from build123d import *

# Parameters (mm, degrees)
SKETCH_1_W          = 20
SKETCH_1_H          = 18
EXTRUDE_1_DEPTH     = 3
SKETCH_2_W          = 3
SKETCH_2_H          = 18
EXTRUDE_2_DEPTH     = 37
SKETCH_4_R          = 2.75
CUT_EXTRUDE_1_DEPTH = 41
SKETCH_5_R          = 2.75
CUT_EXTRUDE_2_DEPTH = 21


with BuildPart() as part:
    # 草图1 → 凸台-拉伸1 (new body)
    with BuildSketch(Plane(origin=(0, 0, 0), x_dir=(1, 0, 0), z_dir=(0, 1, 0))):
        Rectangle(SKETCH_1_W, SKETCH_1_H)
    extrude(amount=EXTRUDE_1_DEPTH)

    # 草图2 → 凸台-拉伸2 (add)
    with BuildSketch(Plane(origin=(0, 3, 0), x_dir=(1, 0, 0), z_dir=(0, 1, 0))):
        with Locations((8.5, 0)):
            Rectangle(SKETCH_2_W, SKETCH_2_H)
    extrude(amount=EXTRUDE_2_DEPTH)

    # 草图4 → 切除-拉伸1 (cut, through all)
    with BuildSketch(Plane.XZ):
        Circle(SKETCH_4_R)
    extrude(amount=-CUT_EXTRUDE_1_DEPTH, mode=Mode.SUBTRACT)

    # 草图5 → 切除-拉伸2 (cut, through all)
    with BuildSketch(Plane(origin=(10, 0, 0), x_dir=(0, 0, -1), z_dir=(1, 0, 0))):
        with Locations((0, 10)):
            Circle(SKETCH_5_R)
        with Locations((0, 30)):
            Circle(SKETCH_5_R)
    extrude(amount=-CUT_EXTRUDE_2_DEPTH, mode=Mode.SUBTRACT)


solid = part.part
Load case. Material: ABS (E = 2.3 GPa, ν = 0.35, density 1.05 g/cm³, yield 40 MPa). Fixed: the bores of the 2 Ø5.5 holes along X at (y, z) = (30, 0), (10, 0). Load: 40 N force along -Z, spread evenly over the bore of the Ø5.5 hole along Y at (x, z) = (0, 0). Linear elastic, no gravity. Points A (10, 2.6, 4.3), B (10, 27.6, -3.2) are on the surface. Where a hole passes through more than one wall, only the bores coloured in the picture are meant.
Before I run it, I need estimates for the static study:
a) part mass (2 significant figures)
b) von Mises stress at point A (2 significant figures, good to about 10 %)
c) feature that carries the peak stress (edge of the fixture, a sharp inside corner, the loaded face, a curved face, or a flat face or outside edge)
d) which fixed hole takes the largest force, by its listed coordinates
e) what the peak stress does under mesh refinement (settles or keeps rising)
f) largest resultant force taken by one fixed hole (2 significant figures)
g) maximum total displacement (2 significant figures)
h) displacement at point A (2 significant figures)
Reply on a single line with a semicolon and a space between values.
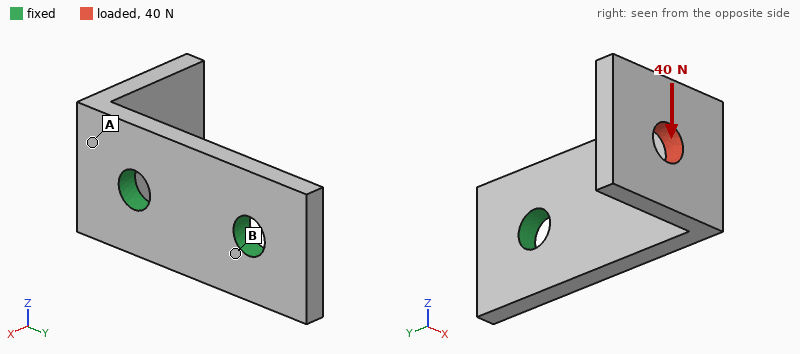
3.0 g; 3.7 MPa; edge of the fixture; (10, 0); keeps rising; 48 N; 0.27 mm; 0.045 mm
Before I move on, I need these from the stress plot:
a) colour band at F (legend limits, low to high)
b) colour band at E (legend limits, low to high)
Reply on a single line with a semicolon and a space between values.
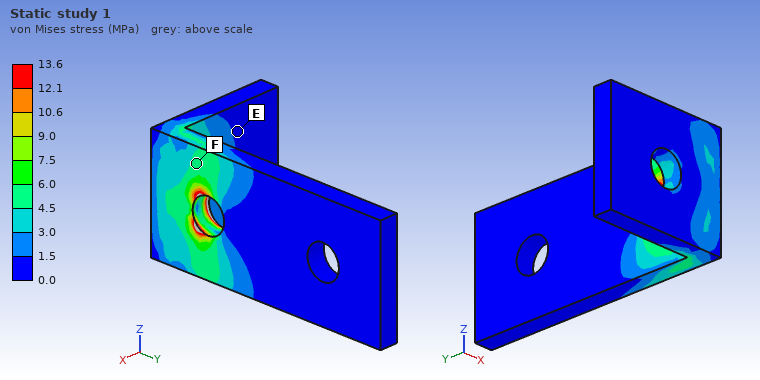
4.5 to 6.0 MPa; 0.0 to 1.5 MPa
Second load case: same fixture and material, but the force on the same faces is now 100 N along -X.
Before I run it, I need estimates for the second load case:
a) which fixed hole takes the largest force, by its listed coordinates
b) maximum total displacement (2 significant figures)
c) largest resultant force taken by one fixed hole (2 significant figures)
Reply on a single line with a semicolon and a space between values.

(10, 0); 0.53 mm; 100 N
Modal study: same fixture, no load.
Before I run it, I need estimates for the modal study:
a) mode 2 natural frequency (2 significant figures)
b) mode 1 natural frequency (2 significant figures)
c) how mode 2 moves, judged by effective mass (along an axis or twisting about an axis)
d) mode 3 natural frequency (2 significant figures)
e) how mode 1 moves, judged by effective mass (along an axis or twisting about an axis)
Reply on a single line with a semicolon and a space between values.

2100 Hz; 1400 Hz; along Z; 4200 Hz; along Y
